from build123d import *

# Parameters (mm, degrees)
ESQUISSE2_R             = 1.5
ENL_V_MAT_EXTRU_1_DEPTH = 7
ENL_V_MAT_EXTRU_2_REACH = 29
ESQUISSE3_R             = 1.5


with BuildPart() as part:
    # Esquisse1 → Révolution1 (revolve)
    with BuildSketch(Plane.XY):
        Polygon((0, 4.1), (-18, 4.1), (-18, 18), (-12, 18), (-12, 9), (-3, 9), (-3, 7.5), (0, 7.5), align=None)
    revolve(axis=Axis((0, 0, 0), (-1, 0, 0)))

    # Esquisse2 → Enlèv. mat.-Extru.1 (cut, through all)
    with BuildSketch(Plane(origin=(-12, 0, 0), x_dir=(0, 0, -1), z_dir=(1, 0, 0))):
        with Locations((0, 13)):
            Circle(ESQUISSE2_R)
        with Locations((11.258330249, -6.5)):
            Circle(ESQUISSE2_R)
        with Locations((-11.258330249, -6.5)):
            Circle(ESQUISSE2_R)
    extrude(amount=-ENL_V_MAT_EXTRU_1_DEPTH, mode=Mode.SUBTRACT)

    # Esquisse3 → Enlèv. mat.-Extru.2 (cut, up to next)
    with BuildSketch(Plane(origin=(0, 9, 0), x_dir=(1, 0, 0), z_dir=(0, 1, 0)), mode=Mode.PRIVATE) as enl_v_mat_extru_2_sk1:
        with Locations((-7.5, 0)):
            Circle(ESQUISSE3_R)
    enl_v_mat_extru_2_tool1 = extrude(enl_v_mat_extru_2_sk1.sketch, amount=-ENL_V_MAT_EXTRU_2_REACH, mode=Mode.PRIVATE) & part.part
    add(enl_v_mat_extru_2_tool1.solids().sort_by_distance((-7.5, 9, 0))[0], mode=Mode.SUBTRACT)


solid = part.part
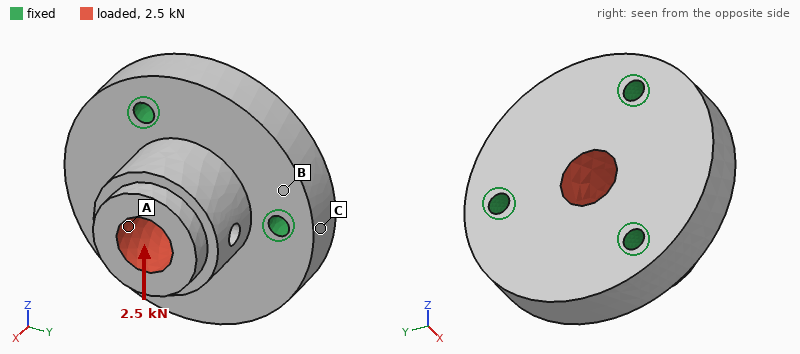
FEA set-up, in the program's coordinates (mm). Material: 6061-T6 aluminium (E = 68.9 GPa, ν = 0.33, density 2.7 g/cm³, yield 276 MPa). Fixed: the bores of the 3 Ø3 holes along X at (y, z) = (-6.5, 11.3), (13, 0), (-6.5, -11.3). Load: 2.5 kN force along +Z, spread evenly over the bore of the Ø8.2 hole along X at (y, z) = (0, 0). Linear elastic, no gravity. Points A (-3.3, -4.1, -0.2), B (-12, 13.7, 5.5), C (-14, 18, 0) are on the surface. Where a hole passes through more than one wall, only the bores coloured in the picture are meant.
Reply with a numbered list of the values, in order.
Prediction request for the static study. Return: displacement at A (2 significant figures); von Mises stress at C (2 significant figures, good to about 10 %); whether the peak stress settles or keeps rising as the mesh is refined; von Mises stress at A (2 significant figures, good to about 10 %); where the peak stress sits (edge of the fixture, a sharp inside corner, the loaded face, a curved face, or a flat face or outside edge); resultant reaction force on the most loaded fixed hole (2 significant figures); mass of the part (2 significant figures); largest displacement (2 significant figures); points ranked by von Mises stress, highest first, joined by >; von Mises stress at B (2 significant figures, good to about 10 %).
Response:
1. 8.6 µm
2. 4.9 MPa
3. keeps rising
4. 20 MPa
5. edge of the fixture
6. 1.1 kN
7. 21 g
8. 12 µm
9. A > B > C
10. 11 MPa
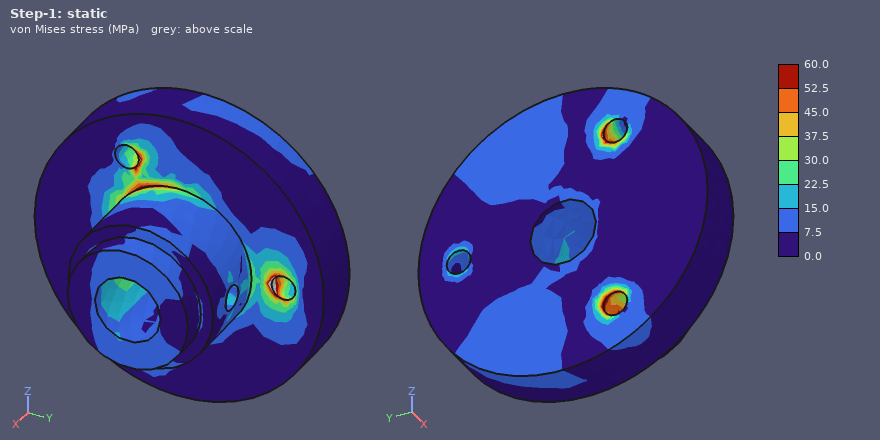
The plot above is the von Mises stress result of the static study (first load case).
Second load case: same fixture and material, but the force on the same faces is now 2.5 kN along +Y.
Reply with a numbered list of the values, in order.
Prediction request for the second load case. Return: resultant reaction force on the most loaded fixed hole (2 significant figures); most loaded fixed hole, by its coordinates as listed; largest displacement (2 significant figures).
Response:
1. 1.2 kN
2. (13, 0)
3. 12 µm
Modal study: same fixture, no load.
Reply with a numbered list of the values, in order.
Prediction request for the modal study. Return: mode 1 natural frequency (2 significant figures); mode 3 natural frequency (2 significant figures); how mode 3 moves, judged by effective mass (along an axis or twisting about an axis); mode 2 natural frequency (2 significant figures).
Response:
1. 25 kHz
2. 30 kHz
3. along X
4. 25 kHz
